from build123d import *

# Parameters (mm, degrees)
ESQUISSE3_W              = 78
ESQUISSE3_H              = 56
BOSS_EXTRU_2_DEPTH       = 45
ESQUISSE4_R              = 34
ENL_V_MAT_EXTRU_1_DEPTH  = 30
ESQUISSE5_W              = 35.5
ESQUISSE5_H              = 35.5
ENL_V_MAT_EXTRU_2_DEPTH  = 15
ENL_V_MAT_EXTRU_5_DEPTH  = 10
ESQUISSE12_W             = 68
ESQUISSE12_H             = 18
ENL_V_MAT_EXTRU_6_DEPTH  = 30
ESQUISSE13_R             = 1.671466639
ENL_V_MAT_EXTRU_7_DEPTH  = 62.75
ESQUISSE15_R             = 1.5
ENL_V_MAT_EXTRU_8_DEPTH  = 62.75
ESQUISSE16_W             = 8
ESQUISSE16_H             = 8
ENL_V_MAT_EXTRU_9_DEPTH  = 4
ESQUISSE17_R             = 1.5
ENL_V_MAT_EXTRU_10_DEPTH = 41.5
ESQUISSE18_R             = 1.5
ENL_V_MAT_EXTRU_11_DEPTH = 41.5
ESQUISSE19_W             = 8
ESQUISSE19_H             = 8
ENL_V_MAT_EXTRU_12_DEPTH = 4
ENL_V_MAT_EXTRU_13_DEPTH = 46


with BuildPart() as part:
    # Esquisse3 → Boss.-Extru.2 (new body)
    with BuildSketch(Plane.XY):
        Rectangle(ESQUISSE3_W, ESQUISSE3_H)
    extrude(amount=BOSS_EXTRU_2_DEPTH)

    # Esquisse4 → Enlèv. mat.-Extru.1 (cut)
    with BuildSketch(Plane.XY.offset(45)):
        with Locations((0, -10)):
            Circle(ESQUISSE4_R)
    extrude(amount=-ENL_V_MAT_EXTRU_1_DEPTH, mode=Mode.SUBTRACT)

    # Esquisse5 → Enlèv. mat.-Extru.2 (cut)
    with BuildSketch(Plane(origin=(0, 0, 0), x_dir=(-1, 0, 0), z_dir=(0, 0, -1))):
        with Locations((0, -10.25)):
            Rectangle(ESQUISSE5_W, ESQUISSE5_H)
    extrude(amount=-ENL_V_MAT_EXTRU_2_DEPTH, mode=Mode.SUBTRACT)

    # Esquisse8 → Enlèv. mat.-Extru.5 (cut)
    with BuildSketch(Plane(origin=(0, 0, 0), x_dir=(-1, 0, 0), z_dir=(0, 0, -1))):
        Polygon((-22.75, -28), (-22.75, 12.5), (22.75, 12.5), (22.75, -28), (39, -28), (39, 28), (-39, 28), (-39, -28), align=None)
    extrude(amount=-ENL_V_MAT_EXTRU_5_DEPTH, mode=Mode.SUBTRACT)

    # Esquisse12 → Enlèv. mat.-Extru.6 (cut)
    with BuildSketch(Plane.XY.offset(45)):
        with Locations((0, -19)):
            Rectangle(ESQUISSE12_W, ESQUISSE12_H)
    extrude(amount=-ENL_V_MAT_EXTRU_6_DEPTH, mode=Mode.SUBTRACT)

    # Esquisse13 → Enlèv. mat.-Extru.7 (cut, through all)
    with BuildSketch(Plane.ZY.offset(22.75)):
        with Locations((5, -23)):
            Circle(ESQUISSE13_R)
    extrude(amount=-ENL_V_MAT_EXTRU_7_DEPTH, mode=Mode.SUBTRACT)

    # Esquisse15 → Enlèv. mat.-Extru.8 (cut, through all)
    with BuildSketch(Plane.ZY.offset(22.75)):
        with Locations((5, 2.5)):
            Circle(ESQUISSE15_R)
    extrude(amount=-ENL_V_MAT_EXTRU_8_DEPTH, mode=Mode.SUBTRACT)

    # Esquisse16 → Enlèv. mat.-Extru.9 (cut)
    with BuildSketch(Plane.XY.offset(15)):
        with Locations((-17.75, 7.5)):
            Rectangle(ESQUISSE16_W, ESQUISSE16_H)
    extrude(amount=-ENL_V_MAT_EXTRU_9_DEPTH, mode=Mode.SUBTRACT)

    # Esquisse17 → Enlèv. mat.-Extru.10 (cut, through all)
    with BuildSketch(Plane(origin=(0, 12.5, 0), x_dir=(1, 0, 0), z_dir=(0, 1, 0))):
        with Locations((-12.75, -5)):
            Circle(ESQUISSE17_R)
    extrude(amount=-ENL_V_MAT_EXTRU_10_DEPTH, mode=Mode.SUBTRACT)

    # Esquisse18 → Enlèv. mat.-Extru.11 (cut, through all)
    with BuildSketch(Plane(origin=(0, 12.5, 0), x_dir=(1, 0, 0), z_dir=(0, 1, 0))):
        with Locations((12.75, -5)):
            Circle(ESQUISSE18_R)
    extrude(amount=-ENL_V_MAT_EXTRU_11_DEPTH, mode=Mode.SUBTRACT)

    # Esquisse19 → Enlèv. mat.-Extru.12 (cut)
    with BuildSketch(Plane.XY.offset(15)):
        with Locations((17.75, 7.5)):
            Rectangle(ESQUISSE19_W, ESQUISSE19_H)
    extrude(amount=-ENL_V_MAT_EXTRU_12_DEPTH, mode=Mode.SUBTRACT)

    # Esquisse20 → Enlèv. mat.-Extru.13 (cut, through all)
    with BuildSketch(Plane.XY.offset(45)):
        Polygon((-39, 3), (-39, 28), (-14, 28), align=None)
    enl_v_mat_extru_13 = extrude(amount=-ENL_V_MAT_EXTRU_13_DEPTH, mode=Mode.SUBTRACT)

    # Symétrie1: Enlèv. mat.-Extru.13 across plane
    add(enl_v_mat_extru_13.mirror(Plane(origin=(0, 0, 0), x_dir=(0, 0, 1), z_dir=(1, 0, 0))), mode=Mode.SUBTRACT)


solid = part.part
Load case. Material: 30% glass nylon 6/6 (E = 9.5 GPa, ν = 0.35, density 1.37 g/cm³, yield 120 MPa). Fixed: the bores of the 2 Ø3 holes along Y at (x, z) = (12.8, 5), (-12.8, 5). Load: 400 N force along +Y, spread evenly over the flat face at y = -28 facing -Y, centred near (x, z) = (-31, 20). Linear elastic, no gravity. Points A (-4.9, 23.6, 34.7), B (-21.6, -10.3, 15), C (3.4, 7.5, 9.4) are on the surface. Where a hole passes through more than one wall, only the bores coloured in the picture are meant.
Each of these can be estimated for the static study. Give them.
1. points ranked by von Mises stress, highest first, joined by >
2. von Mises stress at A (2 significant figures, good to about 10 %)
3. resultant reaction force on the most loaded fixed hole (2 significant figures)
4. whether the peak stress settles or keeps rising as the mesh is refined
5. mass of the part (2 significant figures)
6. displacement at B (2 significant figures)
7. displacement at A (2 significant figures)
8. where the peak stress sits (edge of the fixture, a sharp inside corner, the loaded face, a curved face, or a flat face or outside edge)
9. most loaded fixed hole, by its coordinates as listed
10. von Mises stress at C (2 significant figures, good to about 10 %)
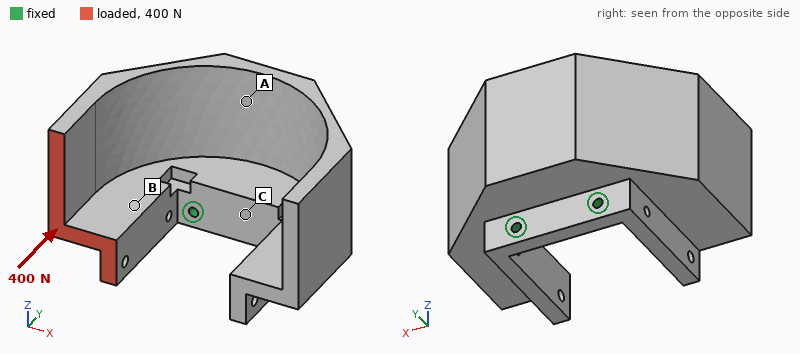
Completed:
C > A > B
6.9 MPa
630 N
keeps rising
53 g
0.42 mm
0.31 mm
edge of the fixture
(-12.8, 5)
13 MPa
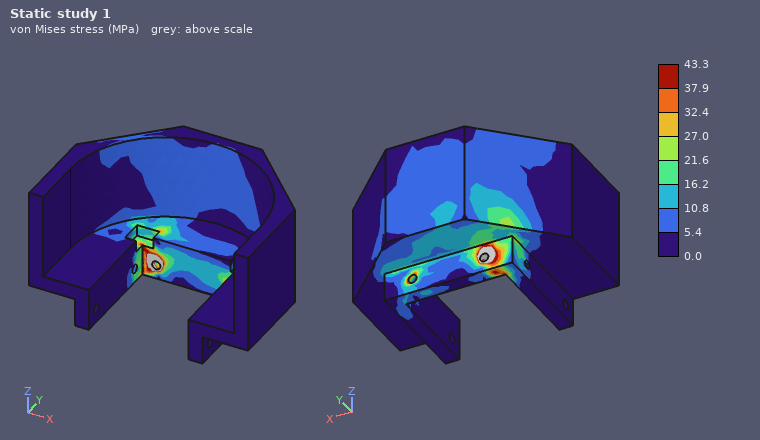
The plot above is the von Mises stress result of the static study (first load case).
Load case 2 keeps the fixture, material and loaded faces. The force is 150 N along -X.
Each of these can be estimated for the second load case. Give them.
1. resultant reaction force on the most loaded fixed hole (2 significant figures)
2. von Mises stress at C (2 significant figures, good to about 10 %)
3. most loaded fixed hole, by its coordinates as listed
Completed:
250 N
7.7 MPa
(-12.8, 5)
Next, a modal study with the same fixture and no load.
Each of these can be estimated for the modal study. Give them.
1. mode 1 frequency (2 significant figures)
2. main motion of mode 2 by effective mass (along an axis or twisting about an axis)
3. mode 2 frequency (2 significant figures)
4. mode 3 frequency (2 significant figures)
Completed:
620 Hz
along X
650 Hz
840 Hz
